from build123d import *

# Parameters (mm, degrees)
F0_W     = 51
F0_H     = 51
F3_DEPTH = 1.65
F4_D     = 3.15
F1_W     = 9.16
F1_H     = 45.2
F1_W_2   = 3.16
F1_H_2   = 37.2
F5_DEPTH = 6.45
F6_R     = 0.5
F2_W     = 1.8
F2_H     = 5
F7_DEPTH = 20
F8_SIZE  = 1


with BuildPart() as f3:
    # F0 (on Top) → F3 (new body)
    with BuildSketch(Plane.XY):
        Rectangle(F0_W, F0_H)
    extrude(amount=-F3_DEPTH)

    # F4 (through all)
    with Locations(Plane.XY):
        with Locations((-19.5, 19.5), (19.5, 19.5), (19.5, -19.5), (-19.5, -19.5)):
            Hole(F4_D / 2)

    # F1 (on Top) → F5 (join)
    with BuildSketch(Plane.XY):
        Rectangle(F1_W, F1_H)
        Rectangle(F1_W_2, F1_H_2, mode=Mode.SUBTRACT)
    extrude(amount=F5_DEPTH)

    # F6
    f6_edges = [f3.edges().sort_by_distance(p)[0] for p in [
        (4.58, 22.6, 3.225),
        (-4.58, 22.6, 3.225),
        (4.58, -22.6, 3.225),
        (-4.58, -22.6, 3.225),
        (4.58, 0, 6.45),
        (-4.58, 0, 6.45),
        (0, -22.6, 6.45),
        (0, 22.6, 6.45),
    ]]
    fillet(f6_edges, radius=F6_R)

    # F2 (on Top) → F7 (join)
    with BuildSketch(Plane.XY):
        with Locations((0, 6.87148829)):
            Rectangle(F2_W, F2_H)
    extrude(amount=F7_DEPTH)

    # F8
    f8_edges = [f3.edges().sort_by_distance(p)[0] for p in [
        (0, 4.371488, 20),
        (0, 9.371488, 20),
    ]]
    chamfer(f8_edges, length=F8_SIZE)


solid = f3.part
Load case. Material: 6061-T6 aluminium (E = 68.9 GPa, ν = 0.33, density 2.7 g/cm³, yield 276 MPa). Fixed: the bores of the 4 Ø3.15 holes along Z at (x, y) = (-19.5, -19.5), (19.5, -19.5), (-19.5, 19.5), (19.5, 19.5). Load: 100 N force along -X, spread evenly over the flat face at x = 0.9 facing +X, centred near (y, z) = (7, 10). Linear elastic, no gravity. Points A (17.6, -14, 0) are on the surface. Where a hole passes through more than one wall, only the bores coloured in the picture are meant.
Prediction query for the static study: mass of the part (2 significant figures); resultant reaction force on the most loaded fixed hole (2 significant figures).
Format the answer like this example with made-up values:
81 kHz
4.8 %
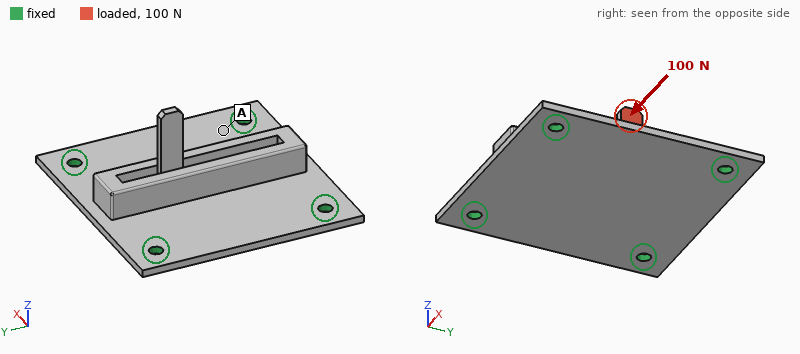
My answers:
17 g
41 N
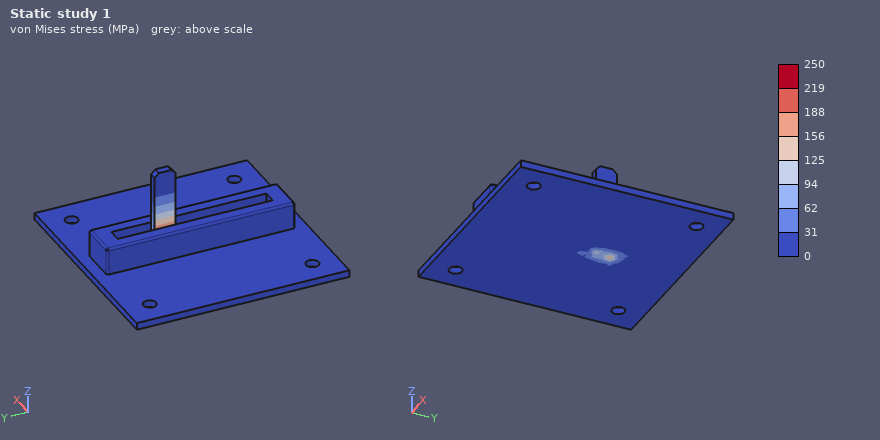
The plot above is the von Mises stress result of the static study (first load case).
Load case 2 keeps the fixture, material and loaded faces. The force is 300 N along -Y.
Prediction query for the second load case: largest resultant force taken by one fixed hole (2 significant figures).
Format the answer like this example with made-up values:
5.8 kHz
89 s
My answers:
100 N
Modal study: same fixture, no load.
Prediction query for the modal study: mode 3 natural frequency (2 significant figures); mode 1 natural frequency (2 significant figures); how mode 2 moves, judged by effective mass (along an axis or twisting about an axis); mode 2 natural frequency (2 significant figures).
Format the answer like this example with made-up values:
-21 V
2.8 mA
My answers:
4900 Hz
3400 Hz
along Z
3600 Hz
